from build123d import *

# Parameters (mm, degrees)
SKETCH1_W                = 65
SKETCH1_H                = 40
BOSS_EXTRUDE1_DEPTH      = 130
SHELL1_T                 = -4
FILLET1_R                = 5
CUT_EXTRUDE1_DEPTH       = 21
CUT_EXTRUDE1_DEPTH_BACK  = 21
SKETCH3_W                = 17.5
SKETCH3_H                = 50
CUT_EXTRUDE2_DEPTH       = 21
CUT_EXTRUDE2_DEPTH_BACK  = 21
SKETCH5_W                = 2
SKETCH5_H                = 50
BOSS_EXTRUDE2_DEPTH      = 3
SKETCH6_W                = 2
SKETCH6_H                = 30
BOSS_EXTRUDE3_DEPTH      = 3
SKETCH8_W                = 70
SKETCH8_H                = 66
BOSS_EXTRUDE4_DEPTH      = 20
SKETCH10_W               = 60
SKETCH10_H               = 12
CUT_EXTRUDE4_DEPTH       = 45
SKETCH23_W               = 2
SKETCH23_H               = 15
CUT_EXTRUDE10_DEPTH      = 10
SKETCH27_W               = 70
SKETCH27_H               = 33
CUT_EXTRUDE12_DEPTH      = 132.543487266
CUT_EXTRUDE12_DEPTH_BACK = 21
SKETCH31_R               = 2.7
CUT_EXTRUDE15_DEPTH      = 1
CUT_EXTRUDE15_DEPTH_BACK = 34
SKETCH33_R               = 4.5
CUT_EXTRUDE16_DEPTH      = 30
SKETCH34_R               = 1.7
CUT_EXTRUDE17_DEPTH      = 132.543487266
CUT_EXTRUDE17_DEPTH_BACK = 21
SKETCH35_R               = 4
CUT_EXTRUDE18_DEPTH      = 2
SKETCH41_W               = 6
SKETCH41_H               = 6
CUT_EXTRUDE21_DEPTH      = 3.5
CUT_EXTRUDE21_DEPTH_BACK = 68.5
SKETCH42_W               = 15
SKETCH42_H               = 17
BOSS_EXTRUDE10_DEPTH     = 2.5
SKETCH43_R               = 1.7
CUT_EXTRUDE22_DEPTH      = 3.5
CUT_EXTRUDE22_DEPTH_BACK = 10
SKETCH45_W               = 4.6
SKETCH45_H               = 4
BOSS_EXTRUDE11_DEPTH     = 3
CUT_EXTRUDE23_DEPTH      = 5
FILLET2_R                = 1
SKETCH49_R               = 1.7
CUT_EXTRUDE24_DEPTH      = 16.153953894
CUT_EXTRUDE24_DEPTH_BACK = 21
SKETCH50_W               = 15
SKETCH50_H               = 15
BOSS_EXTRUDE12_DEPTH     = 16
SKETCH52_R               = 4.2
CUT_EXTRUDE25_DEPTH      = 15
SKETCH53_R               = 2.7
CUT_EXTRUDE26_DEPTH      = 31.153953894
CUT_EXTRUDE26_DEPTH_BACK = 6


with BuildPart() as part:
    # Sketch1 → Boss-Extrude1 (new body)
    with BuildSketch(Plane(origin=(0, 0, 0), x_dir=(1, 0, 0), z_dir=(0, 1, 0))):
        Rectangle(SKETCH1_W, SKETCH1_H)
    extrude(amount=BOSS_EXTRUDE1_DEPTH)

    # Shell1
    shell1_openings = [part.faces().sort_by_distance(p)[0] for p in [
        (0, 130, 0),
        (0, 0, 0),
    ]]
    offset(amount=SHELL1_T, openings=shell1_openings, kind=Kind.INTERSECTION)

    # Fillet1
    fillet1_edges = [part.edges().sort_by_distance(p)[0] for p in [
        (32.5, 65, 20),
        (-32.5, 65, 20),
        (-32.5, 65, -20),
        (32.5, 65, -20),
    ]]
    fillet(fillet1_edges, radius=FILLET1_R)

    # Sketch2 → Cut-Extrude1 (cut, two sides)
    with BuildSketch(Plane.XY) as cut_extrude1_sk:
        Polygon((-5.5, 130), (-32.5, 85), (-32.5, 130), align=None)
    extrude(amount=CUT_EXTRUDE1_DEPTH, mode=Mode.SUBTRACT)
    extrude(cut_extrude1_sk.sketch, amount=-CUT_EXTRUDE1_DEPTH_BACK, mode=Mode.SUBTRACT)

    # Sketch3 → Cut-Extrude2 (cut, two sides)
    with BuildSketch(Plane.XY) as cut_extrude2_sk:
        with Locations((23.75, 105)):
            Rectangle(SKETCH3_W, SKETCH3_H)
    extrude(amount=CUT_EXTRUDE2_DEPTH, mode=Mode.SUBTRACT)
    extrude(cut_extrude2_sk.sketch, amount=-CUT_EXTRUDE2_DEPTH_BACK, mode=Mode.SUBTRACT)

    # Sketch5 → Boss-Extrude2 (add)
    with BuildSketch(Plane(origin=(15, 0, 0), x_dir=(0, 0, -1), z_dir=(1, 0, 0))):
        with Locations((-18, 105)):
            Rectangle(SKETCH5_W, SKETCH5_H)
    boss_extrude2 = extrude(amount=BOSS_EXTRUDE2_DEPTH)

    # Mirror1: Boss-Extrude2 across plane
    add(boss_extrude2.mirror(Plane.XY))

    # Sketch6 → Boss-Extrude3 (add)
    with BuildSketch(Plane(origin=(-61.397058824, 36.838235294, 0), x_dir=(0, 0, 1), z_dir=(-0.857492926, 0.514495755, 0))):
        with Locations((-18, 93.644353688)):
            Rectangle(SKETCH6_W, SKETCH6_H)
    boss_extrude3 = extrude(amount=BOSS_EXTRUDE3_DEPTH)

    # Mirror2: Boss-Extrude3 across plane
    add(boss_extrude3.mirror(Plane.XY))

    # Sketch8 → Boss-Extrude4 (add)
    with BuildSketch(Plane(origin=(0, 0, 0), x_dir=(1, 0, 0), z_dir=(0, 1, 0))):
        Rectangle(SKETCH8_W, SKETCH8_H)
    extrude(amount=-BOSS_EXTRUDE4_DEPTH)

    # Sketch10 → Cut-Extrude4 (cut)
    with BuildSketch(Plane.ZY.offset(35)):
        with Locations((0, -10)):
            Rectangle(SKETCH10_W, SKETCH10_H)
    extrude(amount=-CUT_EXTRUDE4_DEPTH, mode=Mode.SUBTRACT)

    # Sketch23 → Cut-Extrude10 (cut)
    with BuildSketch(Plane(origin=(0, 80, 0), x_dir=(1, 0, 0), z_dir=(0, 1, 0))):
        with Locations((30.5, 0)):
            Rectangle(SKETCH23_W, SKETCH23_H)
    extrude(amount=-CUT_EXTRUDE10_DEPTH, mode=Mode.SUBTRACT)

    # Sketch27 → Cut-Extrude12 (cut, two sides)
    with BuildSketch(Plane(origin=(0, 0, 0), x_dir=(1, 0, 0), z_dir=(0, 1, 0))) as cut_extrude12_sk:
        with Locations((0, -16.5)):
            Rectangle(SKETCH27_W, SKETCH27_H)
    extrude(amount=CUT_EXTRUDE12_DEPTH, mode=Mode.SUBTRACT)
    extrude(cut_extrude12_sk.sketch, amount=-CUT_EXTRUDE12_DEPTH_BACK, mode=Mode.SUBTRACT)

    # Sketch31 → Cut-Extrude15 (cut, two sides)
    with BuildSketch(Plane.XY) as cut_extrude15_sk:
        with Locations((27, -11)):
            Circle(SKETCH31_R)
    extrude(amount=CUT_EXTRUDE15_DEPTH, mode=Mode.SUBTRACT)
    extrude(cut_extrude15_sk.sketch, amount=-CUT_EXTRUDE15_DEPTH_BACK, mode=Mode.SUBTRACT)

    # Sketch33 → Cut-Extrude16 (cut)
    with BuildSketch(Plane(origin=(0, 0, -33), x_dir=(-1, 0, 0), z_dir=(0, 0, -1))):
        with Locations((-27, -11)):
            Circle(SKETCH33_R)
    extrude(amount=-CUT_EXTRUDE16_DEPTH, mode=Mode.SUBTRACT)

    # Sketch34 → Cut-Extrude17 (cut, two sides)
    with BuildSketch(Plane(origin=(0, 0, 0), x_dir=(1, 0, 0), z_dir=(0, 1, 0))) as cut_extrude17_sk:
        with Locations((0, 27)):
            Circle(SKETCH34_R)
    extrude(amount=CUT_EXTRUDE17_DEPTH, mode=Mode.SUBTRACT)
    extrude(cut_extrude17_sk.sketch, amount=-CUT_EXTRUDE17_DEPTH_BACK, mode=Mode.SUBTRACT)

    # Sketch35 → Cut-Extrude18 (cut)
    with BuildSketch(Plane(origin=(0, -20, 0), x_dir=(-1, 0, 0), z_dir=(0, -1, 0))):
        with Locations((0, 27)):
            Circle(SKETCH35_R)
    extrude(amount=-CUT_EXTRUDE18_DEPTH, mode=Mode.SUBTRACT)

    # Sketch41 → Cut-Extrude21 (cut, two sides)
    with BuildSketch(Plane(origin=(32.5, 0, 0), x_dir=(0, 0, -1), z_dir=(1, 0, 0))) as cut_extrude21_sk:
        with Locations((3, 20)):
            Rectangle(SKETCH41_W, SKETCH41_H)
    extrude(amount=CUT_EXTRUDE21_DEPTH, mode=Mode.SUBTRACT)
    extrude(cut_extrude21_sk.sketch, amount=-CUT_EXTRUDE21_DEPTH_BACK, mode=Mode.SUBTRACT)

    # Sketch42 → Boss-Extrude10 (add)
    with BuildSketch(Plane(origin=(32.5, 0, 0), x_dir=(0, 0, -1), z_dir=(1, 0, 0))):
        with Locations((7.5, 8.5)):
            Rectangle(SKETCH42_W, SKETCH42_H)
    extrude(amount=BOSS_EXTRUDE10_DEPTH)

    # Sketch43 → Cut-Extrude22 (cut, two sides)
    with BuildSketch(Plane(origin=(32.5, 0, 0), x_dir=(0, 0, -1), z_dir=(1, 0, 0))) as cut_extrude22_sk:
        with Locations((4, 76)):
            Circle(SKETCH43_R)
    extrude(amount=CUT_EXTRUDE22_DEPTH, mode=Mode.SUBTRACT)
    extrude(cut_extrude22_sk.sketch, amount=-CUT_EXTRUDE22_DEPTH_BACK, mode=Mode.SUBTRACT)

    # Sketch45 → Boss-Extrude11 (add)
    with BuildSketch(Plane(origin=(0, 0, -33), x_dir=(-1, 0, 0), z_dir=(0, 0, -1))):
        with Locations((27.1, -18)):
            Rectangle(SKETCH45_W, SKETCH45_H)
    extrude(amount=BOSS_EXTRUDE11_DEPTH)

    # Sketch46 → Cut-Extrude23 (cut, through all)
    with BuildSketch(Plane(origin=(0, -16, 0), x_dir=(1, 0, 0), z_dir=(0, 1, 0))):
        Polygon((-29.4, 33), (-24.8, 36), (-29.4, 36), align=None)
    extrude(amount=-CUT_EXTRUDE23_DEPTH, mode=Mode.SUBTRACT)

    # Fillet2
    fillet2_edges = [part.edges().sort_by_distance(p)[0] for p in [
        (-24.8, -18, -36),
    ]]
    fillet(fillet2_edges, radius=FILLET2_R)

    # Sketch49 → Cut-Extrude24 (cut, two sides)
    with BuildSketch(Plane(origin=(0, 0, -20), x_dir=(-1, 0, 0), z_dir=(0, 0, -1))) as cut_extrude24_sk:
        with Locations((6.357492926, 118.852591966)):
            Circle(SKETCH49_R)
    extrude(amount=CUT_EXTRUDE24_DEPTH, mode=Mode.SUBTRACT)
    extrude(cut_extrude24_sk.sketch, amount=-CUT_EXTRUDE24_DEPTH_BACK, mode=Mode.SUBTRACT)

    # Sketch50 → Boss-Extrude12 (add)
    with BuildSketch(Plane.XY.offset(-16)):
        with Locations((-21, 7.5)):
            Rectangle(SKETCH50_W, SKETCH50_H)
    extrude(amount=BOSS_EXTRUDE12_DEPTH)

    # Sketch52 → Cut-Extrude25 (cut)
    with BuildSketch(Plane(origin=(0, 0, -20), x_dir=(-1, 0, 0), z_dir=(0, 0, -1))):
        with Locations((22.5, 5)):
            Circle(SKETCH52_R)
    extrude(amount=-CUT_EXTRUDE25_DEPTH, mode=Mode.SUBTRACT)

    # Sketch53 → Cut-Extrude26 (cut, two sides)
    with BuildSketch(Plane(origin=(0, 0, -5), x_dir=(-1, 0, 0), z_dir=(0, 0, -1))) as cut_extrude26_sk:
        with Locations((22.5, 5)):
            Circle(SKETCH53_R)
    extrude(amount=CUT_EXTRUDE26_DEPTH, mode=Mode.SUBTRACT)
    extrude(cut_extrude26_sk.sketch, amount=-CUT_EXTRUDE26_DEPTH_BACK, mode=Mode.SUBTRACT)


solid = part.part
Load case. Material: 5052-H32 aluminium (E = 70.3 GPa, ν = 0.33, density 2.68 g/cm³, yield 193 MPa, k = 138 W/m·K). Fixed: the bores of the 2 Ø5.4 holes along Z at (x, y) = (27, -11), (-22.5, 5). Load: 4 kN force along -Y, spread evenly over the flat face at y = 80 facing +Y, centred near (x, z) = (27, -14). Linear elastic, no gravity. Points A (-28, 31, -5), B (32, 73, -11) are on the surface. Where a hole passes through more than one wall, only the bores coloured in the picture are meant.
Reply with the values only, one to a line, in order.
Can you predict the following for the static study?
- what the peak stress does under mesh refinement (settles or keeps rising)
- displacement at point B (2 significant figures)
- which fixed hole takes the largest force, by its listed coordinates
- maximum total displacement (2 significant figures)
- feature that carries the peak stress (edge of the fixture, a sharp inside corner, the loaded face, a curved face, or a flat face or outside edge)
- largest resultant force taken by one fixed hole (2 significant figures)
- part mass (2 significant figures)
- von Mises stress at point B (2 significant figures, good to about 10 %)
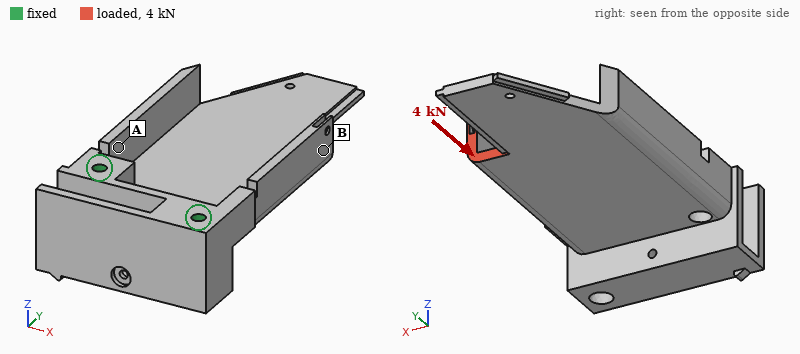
keeps rising
0.50 mm
(27, -11)
0.63 mm
edge of the fixture
3.4 kN
180 g
39 MPa
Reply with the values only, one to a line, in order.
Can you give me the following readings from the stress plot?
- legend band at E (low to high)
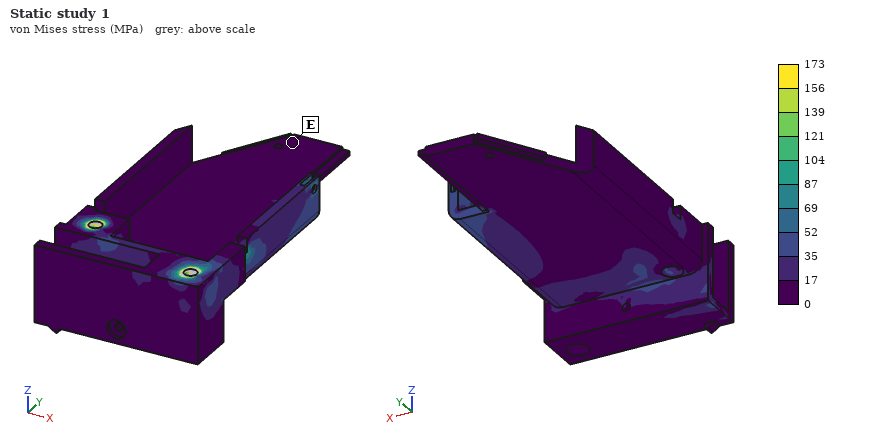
0 to 17 MPa
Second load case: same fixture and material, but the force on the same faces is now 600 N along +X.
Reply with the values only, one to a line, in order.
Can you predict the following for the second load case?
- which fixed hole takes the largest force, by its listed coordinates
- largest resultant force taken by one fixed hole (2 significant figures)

(-22.5, 5)
1.1 kN
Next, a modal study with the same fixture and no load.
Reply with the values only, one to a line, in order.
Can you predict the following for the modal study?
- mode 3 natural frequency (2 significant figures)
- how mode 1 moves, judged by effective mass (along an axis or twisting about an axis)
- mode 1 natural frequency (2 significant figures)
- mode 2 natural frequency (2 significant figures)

1600 Hz
along Z
600 Hz
1300 Hz
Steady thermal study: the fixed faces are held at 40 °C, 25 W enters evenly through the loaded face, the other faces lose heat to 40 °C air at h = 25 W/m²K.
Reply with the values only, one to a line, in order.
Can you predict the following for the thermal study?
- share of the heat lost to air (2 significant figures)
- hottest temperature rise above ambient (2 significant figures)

40 %
60 K
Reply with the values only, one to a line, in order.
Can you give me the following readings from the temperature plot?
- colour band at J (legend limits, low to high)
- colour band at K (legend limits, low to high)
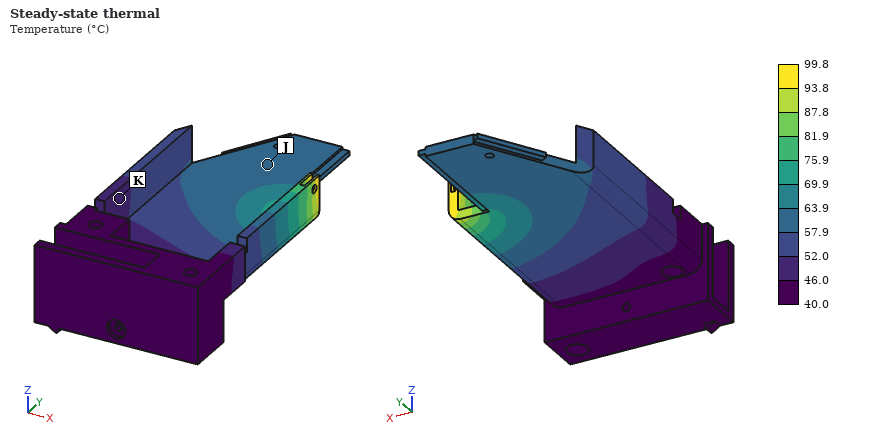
57.9 to 63.9 °C
46.0 to 52.0 °C
